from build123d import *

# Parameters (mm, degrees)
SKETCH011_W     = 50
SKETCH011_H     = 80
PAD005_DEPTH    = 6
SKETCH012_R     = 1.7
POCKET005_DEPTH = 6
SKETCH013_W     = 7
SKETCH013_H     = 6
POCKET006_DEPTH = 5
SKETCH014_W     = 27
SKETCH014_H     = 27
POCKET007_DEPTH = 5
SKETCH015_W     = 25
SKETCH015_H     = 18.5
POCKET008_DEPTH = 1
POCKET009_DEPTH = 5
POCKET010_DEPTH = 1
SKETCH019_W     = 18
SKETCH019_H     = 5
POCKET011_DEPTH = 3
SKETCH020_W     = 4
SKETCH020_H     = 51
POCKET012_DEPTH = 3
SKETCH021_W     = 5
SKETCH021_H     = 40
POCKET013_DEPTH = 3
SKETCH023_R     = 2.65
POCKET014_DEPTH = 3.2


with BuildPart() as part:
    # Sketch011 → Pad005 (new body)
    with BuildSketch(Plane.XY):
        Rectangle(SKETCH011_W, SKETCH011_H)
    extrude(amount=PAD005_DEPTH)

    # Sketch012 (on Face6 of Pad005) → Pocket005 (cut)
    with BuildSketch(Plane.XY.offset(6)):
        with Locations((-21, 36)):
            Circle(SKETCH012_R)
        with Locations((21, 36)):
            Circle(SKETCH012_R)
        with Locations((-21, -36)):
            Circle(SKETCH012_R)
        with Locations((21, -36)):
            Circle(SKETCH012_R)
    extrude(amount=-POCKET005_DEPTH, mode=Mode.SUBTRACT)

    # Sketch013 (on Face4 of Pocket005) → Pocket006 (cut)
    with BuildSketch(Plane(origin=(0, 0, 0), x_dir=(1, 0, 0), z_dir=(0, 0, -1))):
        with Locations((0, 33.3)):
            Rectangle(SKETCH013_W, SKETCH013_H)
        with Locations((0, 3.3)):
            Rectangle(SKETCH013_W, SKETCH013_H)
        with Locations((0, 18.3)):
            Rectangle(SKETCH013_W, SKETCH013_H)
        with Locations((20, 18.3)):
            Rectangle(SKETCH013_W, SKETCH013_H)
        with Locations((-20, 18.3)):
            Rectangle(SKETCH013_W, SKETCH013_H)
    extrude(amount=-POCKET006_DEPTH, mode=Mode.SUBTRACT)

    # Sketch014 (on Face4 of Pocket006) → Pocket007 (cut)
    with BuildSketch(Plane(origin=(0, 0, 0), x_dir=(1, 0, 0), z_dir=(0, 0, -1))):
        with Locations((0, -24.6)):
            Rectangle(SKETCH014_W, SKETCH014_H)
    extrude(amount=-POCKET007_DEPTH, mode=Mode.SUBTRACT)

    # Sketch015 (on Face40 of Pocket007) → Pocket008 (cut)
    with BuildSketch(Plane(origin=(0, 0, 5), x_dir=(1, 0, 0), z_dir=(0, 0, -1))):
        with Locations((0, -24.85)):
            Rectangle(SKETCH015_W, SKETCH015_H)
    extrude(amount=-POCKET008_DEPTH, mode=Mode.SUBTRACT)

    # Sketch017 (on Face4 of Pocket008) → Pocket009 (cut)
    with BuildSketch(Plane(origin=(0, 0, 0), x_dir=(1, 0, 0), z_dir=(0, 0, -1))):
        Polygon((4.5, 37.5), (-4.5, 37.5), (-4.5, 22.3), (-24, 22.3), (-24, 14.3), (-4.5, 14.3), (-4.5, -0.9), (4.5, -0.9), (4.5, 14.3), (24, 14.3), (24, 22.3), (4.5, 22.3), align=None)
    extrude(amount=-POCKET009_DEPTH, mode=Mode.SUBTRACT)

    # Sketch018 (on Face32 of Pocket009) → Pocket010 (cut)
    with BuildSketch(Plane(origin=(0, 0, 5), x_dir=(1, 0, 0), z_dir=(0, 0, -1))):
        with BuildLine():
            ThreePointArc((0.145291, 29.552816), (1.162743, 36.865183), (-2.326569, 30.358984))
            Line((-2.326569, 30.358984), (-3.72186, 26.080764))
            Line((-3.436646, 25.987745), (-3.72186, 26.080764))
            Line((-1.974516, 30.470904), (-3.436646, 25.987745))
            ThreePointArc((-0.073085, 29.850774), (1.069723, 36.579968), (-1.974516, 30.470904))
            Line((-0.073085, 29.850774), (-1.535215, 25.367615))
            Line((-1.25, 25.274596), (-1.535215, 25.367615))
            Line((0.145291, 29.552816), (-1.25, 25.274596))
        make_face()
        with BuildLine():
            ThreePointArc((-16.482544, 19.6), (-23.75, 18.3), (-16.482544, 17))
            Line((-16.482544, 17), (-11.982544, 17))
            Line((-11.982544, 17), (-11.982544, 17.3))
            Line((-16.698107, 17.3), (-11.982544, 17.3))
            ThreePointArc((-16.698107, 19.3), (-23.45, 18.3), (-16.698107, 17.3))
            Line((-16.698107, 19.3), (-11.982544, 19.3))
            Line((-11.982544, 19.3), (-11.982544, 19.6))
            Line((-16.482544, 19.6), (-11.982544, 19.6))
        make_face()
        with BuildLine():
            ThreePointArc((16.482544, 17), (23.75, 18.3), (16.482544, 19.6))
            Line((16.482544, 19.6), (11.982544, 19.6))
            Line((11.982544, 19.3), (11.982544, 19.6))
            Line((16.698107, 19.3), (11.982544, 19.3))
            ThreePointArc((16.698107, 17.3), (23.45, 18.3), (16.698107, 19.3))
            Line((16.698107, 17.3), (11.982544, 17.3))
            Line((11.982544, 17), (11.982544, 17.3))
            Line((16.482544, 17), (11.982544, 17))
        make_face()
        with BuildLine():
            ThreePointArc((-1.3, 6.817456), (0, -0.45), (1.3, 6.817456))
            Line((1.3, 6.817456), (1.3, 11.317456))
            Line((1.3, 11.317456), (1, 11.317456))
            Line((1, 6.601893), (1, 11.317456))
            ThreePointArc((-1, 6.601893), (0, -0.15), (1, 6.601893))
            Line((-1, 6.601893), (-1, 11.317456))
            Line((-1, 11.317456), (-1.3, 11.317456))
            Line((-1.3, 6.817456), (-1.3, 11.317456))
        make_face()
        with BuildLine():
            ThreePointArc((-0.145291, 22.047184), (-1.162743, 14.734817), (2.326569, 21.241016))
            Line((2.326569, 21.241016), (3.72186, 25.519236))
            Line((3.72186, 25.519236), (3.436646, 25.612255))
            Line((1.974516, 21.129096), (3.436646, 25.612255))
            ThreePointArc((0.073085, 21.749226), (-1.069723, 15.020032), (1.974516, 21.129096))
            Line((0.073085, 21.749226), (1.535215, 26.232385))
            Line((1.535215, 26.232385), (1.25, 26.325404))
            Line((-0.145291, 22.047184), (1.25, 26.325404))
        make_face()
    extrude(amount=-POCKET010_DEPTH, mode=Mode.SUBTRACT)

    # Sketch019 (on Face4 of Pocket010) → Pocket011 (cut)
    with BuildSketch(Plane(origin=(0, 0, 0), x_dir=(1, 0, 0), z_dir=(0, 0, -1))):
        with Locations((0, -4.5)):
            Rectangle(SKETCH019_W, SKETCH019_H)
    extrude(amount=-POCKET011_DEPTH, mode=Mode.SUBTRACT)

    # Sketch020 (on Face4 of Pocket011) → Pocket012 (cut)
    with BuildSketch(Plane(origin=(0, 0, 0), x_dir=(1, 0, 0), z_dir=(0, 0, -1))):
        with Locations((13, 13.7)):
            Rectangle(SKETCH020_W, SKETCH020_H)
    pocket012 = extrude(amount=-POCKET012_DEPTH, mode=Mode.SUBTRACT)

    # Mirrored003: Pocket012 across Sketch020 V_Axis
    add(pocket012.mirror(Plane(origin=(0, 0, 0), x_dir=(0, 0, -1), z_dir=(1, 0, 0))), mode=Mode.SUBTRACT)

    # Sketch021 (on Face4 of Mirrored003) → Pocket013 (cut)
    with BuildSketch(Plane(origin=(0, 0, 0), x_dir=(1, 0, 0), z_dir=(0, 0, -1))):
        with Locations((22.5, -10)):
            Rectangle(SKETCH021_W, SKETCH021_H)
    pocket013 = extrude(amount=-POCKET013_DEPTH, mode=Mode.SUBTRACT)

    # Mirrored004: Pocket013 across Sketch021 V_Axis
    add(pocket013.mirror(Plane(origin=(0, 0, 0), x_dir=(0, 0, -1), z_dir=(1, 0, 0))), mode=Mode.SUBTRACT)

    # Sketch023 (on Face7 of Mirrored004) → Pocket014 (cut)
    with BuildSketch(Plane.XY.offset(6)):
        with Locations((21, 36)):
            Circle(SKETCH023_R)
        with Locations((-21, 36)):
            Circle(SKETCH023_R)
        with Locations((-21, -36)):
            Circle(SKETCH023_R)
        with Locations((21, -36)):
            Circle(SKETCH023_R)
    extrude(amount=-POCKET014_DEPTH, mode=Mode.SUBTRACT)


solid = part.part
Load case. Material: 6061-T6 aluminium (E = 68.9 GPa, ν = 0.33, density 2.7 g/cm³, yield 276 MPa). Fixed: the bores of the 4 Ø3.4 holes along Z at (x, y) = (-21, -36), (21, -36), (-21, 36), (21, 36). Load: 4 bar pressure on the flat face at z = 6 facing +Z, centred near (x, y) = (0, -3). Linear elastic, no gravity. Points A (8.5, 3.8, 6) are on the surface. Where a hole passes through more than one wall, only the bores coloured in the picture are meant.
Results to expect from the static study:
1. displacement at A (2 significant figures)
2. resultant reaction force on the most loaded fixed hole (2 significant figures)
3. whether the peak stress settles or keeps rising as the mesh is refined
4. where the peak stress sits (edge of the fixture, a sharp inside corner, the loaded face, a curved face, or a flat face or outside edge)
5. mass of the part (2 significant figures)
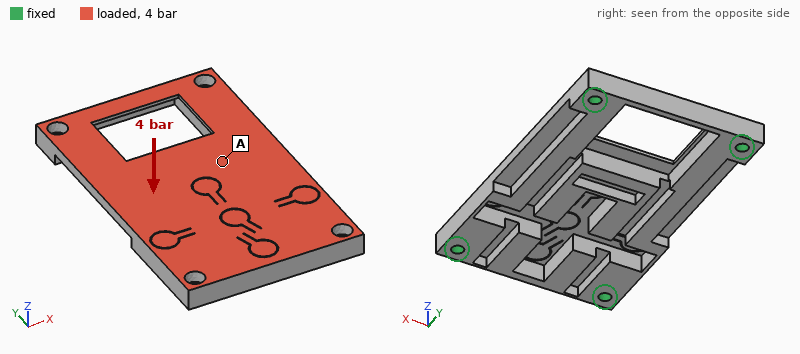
0.11 mm
590 N
keeps rising
a sharp inside corner
37 g
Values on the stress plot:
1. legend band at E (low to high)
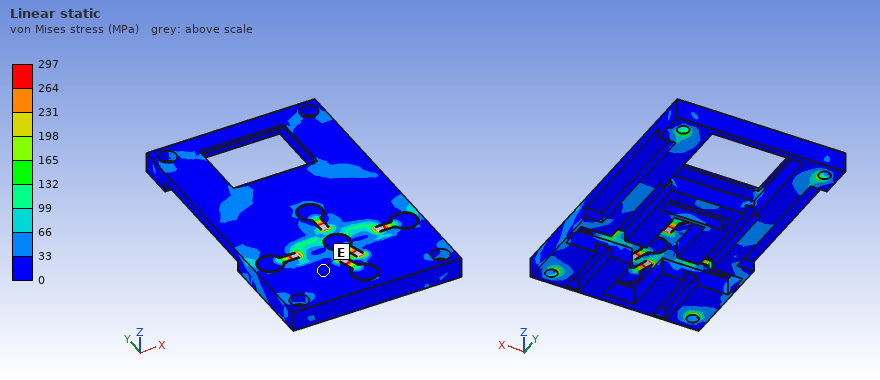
0 to 33 MPa
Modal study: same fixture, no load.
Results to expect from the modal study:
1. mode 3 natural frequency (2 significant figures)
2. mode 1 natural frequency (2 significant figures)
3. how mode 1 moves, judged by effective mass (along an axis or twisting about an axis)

3200 Hz
3100 Hz
along Z
